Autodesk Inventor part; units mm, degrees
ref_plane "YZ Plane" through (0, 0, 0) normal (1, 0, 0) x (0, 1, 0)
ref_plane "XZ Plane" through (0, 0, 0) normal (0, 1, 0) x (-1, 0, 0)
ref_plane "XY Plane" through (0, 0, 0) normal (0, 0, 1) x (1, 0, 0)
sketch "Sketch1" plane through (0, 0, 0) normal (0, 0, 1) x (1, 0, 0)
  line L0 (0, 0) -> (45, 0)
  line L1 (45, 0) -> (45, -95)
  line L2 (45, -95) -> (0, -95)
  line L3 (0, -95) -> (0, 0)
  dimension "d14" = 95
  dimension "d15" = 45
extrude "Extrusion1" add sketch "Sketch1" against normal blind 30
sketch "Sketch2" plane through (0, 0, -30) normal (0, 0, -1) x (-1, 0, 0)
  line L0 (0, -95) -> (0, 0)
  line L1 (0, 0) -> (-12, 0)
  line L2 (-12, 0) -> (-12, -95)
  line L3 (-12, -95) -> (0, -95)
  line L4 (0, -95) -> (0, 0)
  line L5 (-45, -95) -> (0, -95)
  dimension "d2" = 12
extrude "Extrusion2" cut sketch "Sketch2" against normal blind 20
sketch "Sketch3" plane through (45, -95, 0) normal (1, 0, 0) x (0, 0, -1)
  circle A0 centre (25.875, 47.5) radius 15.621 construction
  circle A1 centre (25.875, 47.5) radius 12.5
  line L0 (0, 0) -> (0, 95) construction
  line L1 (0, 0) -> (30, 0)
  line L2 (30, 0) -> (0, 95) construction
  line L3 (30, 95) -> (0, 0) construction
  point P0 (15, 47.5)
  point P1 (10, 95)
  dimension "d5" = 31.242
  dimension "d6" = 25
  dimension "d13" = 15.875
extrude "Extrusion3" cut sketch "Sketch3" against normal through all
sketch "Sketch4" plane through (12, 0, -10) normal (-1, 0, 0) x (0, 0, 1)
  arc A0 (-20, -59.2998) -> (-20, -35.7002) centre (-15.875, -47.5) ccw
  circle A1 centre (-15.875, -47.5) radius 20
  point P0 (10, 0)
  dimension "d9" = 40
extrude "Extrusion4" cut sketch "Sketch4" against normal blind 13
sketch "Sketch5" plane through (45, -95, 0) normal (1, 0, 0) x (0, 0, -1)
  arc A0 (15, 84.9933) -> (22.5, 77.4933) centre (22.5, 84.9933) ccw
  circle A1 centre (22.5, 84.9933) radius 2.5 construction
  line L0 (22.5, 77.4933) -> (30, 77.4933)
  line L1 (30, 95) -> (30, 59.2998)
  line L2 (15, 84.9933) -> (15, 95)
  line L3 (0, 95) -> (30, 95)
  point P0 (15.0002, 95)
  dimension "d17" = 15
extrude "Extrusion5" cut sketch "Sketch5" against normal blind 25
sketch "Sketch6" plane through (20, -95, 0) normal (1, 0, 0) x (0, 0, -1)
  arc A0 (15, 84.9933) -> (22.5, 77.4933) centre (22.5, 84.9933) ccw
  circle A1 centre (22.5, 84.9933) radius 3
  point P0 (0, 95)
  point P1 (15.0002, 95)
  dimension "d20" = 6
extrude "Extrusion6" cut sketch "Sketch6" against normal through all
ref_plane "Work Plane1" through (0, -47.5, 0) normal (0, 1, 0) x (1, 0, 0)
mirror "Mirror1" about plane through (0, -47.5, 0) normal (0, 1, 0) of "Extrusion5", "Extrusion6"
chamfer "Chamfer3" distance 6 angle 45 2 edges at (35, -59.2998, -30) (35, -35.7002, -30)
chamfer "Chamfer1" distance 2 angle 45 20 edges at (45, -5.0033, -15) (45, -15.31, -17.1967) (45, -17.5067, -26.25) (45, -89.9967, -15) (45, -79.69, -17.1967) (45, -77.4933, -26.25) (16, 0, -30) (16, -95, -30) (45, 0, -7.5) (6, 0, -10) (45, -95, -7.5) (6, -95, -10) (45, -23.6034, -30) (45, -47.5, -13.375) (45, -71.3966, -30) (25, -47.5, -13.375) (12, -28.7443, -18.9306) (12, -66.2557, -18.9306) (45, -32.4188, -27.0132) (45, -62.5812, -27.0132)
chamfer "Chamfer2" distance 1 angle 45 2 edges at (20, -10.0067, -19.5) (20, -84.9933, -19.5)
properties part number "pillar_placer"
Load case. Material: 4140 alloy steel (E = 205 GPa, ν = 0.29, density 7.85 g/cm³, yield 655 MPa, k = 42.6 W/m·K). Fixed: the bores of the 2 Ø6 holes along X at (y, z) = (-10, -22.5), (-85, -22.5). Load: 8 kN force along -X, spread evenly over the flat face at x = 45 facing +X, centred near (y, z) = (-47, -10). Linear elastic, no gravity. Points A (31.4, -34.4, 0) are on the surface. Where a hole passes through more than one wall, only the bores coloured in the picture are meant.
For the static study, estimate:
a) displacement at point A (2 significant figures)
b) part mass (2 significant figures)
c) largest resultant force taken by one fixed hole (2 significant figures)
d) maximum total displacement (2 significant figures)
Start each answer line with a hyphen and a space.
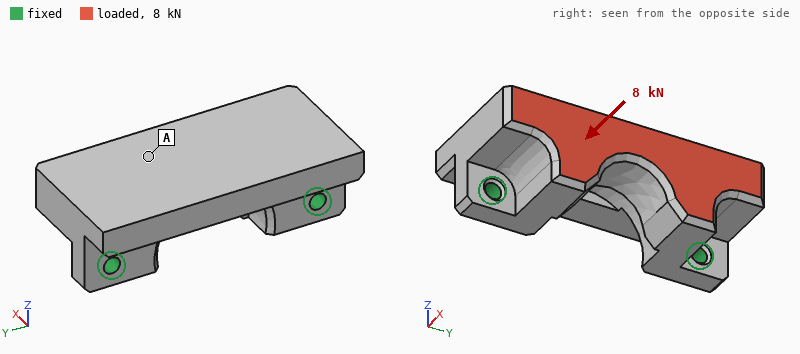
- 36 µm
- 580 g
- 4.0 kN
- 48 µm
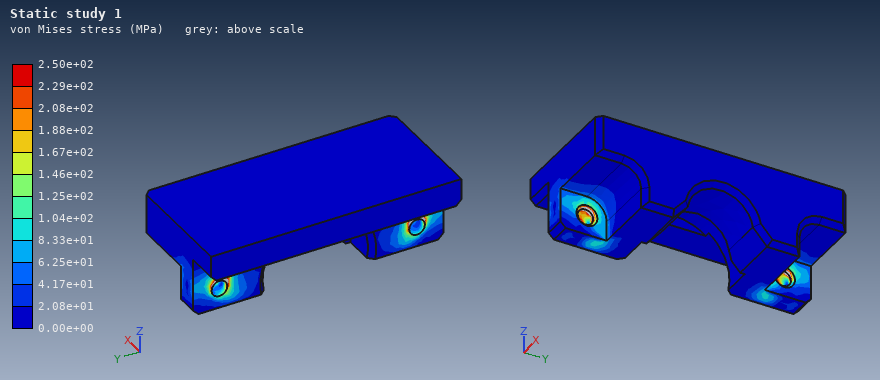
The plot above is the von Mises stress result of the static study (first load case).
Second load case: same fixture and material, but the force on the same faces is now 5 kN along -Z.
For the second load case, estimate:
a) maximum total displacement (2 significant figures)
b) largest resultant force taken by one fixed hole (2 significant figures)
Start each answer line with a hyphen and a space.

- 84 µm
- 2.9 kN
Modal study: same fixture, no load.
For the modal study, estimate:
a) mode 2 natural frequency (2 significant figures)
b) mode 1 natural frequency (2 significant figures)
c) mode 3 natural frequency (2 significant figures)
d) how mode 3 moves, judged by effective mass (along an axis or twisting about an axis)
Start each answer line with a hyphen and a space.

- 6400 Hz
- 2700 Hz
- 9500 Hz
- along Y
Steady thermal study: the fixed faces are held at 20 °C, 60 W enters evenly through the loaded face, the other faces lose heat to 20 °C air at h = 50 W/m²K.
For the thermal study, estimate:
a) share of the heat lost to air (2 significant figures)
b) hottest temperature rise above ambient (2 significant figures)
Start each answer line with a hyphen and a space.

- 32 %
- 47 K
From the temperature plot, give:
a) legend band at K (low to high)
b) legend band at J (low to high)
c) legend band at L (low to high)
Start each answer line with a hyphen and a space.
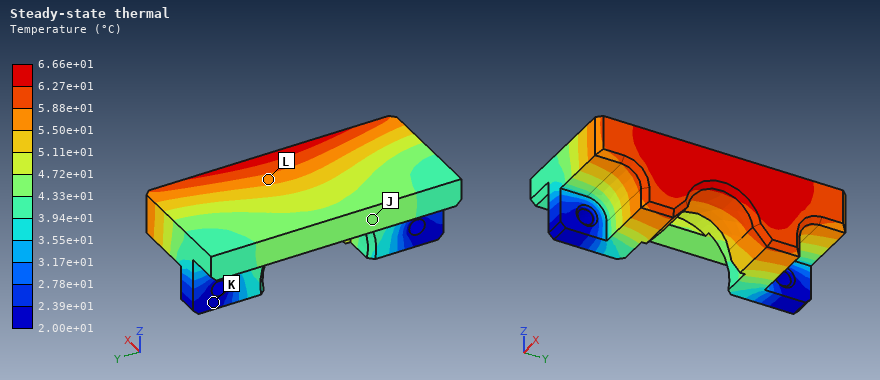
- 2.00e+01 to 2.39e+01 °C
- 4.33e+01 to 4.72e+01 °C
- 5.50e+01 to 5.88e+01 °C
